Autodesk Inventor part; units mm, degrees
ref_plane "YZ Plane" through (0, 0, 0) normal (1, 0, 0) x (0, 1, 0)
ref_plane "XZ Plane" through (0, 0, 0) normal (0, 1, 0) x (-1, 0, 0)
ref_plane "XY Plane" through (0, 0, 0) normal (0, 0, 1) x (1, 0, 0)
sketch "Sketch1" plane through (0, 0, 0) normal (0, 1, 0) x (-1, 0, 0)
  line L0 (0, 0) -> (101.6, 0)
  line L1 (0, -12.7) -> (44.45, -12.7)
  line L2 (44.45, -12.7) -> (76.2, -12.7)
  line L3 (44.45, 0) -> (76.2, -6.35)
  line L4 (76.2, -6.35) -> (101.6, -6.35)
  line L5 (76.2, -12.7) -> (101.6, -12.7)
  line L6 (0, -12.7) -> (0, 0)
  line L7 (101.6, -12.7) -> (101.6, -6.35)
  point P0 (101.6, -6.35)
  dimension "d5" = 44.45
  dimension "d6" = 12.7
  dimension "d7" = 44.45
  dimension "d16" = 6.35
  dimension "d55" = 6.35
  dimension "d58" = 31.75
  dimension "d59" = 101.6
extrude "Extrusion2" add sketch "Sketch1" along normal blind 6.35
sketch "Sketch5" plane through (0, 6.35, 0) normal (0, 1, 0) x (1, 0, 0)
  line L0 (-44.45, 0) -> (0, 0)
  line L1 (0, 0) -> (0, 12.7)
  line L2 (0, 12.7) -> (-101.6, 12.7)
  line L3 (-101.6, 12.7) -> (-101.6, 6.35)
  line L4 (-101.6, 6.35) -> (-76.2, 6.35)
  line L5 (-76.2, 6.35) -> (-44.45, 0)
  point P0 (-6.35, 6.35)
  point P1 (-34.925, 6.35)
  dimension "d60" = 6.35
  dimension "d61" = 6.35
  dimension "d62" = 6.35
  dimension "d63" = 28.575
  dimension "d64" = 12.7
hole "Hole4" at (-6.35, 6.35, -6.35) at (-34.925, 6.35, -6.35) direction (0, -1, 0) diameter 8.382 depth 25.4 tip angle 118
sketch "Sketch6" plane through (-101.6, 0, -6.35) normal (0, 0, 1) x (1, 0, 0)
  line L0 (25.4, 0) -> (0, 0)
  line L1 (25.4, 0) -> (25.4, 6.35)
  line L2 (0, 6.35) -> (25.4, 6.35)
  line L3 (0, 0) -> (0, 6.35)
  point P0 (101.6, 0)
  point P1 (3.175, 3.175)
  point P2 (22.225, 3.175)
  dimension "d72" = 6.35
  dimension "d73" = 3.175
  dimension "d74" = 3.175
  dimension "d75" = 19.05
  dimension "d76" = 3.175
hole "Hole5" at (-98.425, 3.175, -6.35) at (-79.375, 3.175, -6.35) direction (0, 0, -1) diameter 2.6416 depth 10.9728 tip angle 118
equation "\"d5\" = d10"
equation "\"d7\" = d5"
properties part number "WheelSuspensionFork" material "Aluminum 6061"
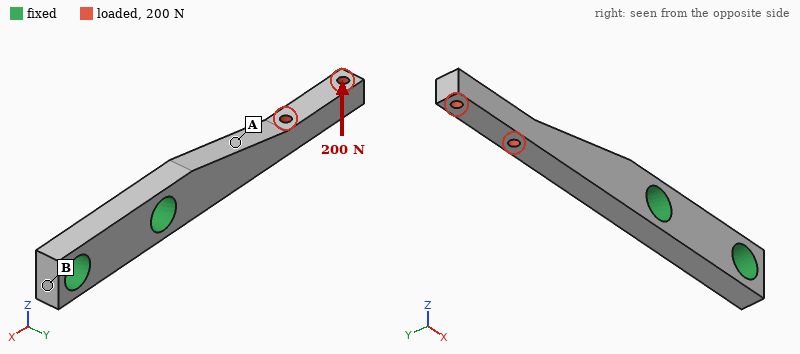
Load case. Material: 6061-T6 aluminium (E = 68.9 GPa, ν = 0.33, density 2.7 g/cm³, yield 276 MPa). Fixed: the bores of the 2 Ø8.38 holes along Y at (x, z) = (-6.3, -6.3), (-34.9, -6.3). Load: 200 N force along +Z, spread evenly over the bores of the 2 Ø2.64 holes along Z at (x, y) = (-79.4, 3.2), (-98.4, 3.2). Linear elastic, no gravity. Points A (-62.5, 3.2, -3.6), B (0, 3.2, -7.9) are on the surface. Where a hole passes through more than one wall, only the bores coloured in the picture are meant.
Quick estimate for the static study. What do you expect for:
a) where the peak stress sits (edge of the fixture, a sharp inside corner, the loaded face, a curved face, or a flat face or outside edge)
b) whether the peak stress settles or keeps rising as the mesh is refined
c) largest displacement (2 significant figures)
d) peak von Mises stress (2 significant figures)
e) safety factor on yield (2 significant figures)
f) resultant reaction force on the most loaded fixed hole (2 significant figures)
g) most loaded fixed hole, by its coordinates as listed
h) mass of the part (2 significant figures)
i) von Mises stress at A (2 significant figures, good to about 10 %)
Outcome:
the loaded face
settles
0.38 mm
130 MPa
2.1
220 N
(-34.9, -6.3)
16 g
62 MPa
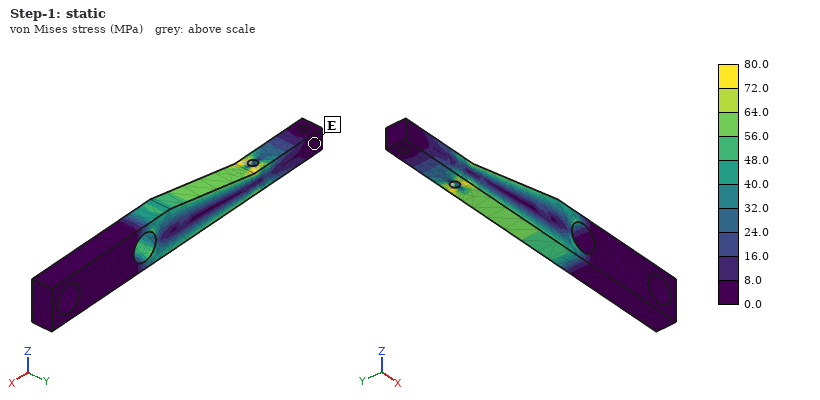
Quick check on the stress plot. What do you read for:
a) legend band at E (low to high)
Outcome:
0.0 to 8.0 MPa
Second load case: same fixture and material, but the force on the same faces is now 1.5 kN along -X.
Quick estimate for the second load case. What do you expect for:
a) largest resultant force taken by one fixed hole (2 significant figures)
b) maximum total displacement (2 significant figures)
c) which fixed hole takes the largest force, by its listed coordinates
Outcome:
1.5 kN
0.12 mm
(-34.9, -6.3)
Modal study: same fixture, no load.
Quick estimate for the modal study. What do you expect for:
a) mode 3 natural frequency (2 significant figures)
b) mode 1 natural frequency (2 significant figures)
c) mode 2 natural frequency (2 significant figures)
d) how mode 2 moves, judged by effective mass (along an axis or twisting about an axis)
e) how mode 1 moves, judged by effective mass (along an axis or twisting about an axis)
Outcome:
8200 Hz
1700 Hz
2600 Hz
along Z
along Y
